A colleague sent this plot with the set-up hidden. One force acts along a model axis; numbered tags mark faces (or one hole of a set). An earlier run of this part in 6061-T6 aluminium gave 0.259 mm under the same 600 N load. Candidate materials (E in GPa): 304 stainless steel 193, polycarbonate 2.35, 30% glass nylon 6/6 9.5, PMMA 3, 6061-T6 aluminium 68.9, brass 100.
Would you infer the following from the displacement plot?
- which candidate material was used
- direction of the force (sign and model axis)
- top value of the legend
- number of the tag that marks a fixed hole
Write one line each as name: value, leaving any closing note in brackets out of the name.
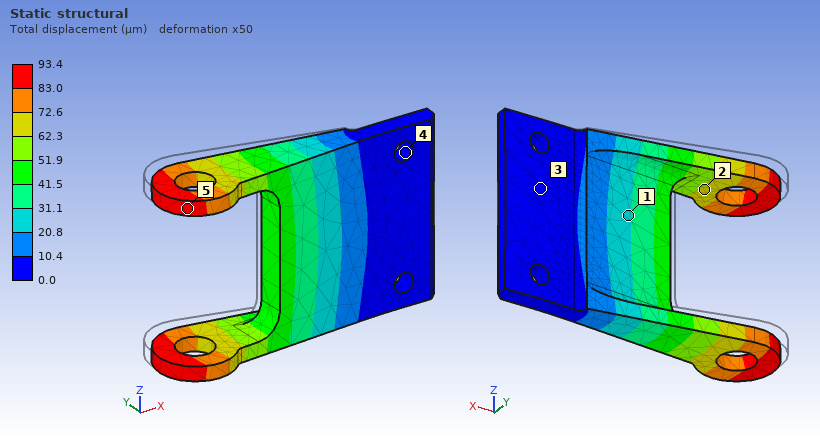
which candidate material was used: 304 stainless steel
direction of the force: -Y
top value of the legend: 93.4 µm
number of the tag that marks a fixed hole: 4
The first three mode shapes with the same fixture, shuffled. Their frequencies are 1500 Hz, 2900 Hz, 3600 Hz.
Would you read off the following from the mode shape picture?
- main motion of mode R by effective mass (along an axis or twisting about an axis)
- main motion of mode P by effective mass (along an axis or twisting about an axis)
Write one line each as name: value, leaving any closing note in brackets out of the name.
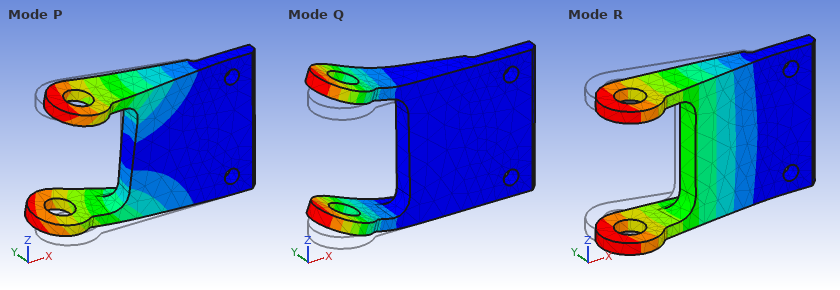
main motion of mode R by effective mass: along Y
main motion of mode P by effective mass: twisting about X
